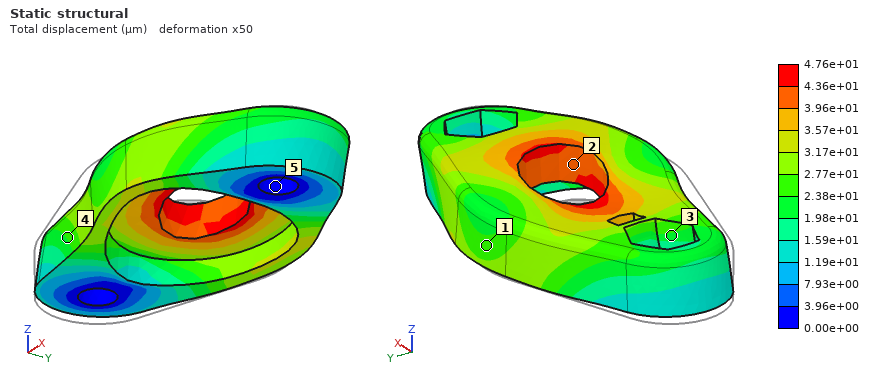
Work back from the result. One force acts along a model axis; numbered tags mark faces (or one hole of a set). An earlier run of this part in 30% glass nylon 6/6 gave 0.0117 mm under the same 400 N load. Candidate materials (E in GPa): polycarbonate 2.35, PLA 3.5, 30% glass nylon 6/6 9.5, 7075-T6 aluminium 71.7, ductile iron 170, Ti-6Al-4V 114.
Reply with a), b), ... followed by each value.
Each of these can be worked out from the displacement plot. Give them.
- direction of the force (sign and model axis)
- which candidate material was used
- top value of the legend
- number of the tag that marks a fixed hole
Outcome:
a) +X
b) polycarbonate
c) 4.76e+01 µm
d) 5
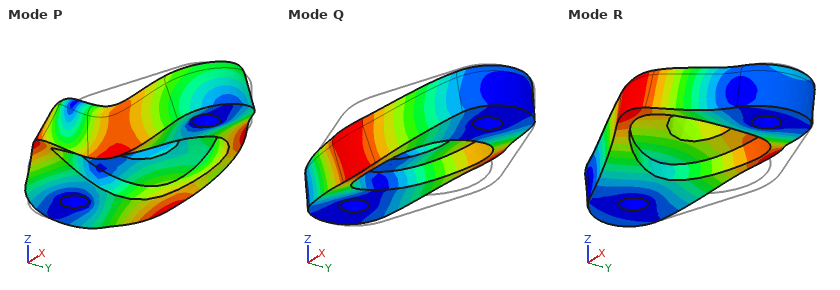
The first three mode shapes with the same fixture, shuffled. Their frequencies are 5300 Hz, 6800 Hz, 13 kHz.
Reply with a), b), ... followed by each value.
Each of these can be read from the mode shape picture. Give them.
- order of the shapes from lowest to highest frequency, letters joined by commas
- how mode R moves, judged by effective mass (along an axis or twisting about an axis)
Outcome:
a) Q, R, P
b) along Z
